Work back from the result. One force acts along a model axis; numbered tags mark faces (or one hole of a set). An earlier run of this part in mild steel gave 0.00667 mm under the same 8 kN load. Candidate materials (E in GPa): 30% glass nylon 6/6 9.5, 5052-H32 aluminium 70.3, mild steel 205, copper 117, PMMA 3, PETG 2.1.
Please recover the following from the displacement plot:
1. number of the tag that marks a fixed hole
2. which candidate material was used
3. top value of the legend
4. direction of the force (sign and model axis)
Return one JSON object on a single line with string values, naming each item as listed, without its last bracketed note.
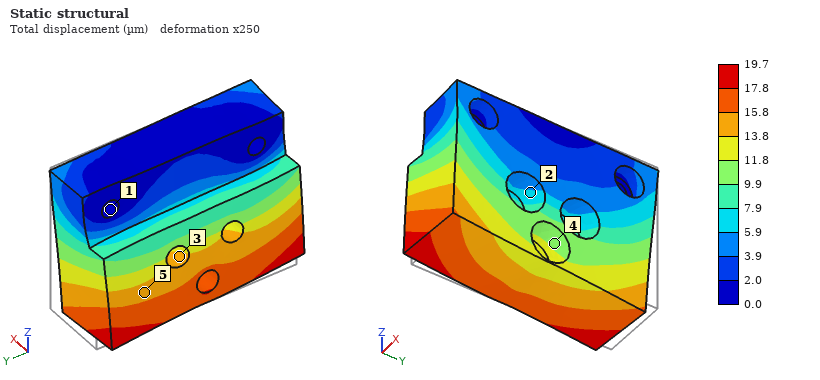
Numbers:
{"number of the tag that marks a fixed hole": "1", "which candidate material was used": "5052-H32 aluminium", "top value of the legend": "19.7 µm", "direction of the force": "-Y"}
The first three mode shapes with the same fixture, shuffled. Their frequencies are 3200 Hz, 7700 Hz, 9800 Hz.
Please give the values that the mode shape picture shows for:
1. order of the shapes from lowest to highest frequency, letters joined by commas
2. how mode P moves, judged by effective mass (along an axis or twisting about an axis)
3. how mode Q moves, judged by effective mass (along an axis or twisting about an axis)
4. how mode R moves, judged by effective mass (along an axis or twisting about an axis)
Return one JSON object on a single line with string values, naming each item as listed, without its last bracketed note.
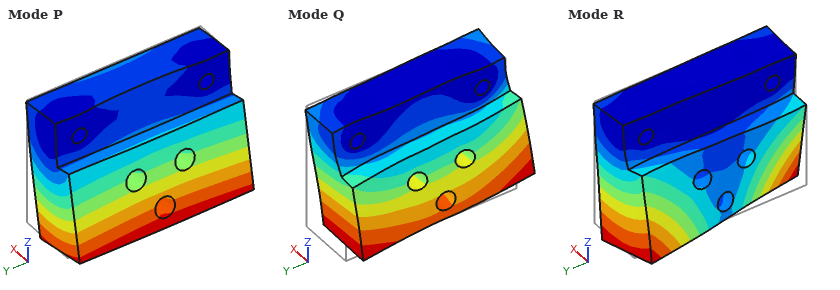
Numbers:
{"order of the shapes from lowest to highest frequency, letters joined by commas": "P, R, Q", "how mode P moves, judged by effective mass": "along X", "how mode Q moves, judged by effective mass": "along Y", "how mode R moves, judged by effective mass": "twisting about Z"}
